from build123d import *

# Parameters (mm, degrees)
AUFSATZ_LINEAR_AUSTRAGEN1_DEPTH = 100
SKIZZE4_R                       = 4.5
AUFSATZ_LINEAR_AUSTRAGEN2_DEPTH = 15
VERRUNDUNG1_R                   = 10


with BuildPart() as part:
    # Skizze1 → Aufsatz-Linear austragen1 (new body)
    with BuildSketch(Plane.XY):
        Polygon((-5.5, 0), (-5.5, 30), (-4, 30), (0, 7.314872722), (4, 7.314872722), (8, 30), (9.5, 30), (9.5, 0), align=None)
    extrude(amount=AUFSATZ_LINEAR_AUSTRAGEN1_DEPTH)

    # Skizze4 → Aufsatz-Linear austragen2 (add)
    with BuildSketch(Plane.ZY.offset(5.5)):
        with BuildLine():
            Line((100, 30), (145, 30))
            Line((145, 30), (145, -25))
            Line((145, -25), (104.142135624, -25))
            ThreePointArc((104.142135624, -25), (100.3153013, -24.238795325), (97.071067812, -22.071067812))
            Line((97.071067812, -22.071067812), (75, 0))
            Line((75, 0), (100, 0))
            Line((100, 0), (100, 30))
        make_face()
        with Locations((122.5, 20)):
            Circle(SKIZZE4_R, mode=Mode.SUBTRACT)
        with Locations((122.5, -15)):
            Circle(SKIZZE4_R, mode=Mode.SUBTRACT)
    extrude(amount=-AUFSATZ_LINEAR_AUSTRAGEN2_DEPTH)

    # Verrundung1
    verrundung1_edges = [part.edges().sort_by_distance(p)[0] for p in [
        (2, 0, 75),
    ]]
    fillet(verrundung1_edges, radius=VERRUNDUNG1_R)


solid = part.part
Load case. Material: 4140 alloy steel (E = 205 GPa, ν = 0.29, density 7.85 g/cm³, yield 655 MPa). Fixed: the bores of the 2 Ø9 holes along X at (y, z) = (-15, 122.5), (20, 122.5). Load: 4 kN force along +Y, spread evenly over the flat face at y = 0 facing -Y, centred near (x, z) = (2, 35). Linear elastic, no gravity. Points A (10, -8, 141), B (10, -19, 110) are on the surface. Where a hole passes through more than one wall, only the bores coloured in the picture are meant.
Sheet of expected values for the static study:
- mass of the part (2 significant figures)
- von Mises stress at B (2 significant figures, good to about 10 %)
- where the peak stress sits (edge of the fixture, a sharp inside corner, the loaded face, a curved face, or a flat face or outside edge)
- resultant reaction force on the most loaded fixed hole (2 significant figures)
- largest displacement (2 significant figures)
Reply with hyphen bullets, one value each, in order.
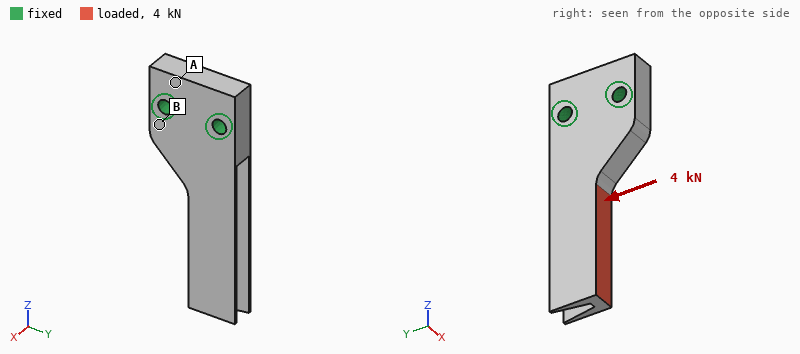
- 520 g
- 30 MPa
- a curved face
- 9.2 kN
- 0.17 mm
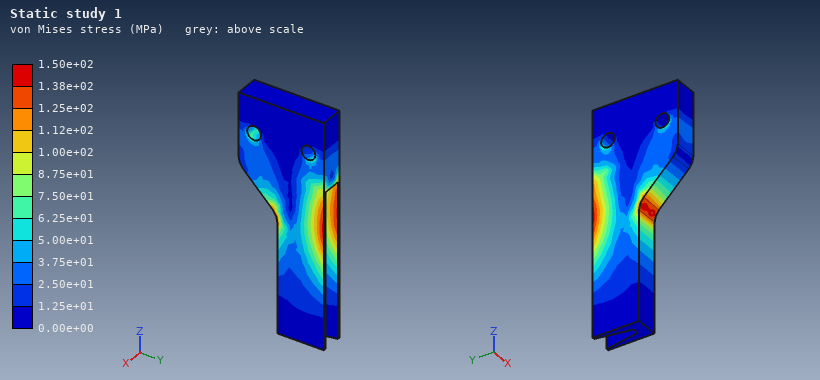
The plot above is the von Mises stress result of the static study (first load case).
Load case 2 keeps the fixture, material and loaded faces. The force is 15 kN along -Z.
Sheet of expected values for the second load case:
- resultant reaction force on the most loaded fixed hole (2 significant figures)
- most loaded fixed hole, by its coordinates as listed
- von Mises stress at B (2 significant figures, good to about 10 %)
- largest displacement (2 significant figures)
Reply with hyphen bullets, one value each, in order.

- 8.7 kN
- (-15, 122.5)
- 20 MPa
- 0.15 mm
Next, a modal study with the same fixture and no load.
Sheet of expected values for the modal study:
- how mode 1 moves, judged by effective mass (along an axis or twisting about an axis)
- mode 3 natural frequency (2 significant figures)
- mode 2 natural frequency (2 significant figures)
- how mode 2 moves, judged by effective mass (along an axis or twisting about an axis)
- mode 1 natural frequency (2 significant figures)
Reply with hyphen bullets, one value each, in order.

- along X
- 3600 Hz
- 2500 Hz
- along Y
- 1100 Hz
